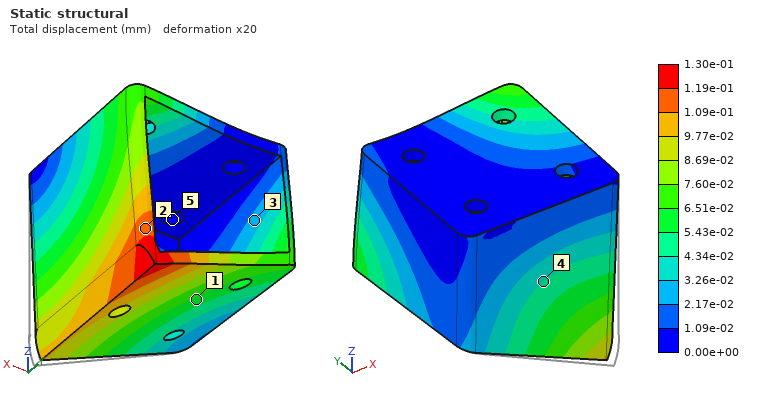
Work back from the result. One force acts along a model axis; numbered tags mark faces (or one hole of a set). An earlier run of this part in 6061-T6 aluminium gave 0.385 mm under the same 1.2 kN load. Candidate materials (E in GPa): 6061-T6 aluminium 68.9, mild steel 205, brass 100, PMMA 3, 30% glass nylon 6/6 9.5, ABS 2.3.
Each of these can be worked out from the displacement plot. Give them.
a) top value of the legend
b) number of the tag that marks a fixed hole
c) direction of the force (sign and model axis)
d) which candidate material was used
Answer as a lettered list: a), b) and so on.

a) 1.30e-01 mm
b) 5
c) +Y
d) mild steel
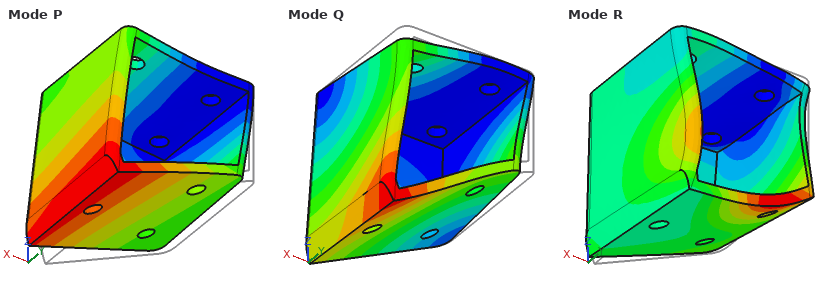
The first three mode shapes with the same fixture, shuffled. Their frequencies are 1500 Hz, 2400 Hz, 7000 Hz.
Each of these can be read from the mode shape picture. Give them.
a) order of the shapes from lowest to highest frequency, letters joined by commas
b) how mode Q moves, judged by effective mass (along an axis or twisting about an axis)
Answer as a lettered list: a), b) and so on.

a) P, Q, R
b) along Y
